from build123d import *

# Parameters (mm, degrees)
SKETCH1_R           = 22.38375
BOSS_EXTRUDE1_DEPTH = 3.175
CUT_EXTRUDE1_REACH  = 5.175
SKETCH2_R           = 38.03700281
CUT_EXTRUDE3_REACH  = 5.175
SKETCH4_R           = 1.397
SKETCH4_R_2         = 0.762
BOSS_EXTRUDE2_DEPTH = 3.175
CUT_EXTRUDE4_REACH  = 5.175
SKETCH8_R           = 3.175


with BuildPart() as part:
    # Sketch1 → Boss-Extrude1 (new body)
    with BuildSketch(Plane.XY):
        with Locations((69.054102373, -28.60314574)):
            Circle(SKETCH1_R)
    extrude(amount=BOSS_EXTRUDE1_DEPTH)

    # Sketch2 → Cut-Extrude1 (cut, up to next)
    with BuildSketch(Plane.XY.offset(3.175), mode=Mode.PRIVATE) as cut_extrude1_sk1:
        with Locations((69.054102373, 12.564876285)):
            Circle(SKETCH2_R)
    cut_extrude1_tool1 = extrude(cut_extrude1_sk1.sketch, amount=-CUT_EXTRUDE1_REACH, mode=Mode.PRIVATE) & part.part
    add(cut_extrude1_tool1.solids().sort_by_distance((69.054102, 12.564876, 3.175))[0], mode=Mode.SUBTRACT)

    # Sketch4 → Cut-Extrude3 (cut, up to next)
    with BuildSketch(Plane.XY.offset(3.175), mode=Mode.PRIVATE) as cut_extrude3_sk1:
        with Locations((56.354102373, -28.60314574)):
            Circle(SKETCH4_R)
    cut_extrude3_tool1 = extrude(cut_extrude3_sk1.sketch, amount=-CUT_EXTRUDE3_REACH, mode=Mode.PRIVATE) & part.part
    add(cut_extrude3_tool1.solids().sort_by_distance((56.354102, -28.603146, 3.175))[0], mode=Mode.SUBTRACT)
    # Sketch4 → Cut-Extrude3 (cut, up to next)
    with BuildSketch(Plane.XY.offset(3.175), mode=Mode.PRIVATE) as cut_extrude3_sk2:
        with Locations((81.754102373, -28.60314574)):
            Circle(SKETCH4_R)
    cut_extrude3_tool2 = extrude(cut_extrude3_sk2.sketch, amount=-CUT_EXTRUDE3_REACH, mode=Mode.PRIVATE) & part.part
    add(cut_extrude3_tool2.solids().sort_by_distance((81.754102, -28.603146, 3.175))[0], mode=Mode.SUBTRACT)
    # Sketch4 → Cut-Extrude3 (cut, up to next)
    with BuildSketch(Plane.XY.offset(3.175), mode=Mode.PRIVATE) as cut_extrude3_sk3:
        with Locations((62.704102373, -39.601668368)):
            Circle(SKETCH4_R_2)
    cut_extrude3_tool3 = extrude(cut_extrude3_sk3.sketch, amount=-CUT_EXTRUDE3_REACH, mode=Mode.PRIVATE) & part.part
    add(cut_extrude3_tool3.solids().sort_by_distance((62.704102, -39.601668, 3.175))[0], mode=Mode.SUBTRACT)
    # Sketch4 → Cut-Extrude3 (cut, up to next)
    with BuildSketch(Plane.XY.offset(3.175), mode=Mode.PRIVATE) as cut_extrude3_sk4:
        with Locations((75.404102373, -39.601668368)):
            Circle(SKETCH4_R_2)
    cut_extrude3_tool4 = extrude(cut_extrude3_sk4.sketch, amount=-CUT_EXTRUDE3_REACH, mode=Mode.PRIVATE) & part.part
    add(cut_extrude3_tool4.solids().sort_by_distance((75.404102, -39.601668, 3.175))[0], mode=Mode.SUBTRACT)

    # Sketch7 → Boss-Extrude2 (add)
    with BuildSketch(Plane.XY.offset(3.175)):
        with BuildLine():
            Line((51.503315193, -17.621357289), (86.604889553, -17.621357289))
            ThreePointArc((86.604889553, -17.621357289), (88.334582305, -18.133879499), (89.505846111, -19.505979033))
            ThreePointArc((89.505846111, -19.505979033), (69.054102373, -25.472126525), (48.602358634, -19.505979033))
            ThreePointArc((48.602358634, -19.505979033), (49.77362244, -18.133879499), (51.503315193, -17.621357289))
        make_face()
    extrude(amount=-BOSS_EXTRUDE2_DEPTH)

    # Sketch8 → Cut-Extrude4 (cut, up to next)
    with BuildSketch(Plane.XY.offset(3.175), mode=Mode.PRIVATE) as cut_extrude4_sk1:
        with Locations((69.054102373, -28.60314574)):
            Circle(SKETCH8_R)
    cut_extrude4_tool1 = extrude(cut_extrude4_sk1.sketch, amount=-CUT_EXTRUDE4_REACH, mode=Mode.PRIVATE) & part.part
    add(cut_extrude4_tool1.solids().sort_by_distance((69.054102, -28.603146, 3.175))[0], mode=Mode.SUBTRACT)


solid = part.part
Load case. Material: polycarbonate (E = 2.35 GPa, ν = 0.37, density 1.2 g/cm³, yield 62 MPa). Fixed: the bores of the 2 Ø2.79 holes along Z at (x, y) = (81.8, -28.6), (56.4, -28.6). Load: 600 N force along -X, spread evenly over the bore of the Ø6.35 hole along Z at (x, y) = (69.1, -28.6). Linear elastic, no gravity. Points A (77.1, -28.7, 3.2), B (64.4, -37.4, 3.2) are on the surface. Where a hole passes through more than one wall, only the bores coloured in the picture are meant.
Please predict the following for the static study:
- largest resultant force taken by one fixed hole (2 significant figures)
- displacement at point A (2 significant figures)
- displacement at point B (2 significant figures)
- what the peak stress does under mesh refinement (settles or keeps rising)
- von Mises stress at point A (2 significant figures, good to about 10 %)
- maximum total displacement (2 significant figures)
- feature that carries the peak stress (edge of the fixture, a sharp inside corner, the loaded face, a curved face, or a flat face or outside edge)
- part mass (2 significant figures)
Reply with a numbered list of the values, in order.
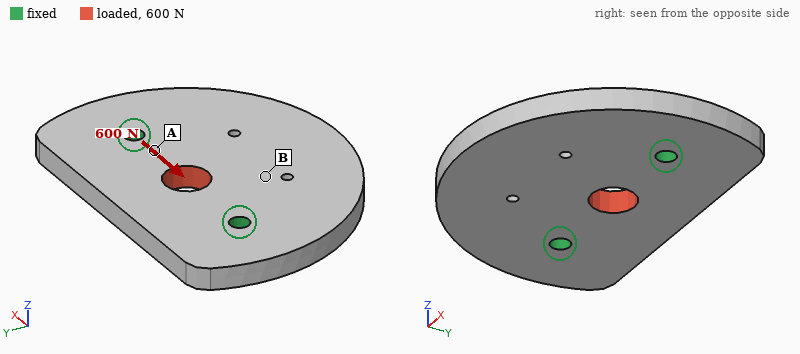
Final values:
1. 300 N
2. 19 µm
3. 23 µm
4. keeps rising
5. 12 MPa
6. 49 µm
7. edge of the fixture
8. 4.6 g
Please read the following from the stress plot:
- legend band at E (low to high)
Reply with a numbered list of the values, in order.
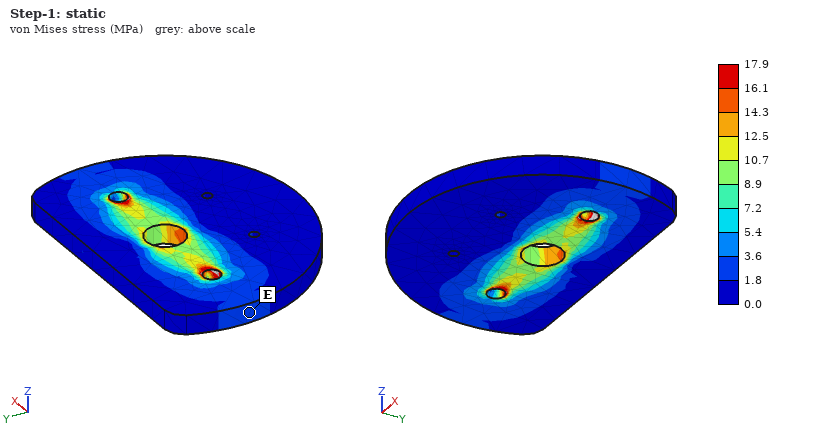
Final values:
1. 1.8 to 3.6 MPa
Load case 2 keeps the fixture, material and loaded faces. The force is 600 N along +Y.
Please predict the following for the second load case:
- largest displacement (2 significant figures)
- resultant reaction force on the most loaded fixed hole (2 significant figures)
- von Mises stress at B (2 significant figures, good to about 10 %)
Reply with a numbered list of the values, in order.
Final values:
1. 86 µm
2. 300 N
3. 5.1 MPa
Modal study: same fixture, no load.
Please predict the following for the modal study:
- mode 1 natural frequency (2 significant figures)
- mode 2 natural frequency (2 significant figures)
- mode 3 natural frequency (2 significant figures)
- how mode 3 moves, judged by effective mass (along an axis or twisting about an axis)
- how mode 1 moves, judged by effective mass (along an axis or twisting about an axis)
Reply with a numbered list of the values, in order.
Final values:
1. 1600 Hz
2. 3400 Hz
3. 4400 Hz
4. along Z
5. along Z
